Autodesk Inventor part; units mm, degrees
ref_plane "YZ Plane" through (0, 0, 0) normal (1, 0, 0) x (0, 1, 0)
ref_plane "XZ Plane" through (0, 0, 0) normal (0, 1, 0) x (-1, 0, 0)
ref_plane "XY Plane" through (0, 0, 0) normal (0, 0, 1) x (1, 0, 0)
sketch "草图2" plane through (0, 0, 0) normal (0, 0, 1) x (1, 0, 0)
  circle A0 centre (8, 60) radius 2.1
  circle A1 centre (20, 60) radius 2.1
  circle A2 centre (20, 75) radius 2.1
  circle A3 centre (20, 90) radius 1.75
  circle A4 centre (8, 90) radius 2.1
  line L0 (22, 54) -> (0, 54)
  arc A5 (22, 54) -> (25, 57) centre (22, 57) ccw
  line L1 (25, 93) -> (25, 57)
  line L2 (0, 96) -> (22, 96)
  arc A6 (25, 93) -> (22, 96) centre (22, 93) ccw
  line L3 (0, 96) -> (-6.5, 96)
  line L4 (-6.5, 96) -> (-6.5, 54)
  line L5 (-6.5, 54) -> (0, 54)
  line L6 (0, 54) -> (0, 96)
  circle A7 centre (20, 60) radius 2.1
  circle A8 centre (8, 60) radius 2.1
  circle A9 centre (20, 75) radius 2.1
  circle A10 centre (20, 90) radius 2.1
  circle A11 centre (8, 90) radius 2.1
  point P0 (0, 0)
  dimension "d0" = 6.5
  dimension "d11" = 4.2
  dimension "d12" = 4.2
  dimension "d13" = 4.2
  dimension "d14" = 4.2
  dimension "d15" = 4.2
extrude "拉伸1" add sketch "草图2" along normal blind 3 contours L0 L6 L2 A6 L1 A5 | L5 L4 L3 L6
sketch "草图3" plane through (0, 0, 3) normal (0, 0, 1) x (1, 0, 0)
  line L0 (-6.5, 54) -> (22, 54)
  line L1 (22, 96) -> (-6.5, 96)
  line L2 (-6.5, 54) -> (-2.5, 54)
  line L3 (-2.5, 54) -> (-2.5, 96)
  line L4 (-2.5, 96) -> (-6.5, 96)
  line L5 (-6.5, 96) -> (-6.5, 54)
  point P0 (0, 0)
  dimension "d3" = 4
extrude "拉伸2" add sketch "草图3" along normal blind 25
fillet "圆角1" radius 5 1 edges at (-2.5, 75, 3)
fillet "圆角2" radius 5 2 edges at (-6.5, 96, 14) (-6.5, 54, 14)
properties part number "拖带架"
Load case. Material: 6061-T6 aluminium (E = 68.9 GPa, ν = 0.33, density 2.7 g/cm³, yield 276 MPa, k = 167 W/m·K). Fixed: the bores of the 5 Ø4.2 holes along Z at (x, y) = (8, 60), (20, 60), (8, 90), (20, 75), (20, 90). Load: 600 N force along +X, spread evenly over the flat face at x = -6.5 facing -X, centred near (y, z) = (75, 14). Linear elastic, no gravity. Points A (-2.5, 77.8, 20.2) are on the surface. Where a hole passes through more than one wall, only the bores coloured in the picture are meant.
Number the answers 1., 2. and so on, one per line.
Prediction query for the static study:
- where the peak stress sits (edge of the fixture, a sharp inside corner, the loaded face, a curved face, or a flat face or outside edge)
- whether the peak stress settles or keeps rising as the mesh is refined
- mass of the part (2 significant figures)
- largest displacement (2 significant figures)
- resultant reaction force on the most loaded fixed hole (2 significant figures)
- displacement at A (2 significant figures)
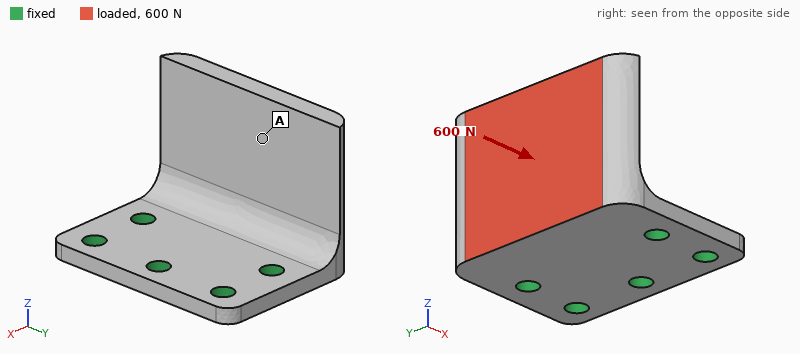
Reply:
1. edge of the fixture
2. keeps rising
3. 21 g
4. 0.32 mm
5. 240 N
6. 0.21 mm
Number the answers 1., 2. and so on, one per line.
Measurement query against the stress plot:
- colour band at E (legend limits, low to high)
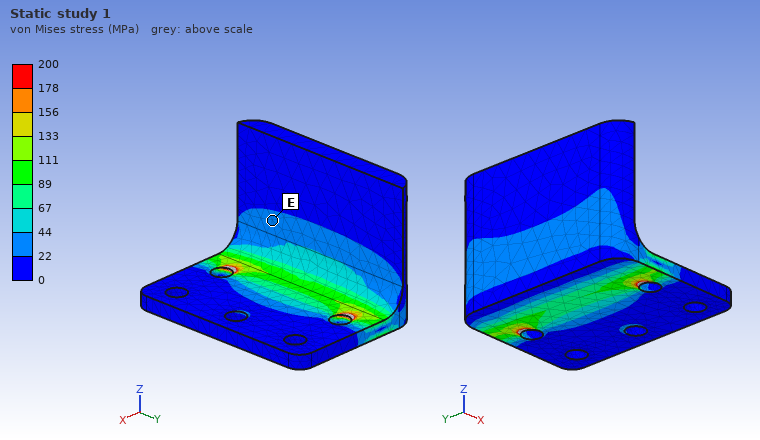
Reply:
1. 22 to 44 MPa
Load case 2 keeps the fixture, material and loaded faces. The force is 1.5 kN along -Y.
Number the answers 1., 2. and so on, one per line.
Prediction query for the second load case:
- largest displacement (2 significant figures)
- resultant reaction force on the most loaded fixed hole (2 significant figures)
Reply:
1. 93 µm
2. 1.1 kN
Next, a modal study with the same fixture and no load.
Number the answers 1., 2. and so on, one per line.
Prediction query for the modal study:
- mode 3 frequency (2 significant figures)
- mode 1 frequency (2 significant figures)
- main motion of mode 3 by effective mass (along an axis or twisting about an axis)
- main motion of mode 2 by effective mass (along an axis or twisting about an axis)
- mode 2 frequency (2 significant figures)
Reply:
1. 8700 Hz
2. 2300 Hz
3. along Z
4. along Y
5. 5400 Hz
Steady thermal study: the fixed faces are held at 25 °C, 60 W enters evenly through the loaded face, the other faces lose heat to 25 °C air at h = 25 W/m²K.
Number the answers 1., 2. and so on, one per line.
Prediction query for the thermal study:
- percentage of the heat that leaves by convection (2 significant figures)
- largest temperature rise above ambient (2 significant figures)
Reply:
1. 4.1 %
2. 57 K
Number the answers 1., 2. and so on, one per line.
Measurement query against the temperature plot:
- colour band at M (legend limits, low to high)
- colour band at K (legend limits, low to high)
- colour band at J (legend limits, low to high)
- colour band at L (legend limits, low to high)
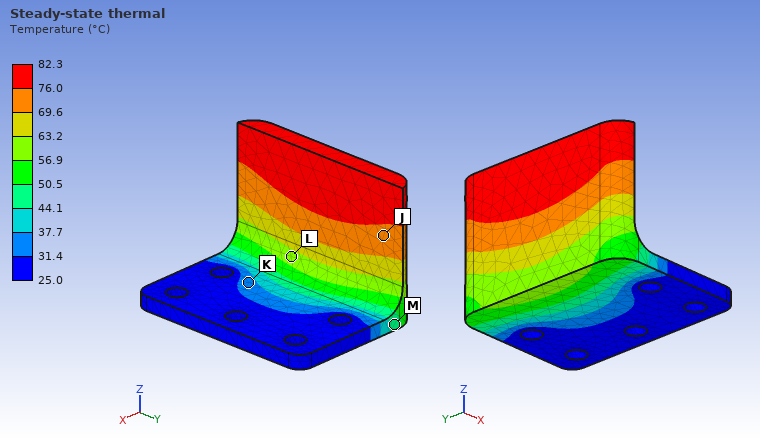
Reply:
1. 44.1 to 50.5 °C
2. 31.4 to 37.7 °C
3. 69.6 to 76.0 °C
4. 56.9 to 63.2 °C
